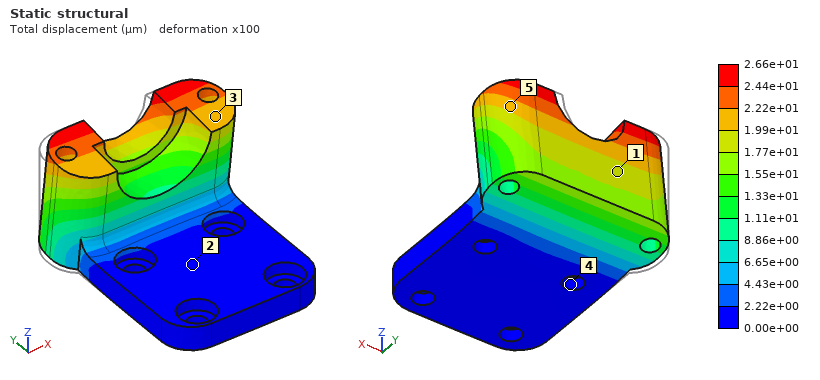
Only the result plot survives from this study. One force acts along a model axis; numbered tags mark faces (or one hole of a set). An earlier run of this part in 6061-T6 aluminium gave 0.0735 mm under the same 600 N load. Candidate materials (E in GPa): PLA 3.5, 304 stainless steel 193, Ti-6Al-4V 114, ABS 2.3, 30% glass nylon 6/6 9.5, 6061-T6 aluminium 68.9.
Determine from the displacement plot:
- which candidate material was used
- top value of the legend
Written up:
304 stainless steel
2.66e+01 µm
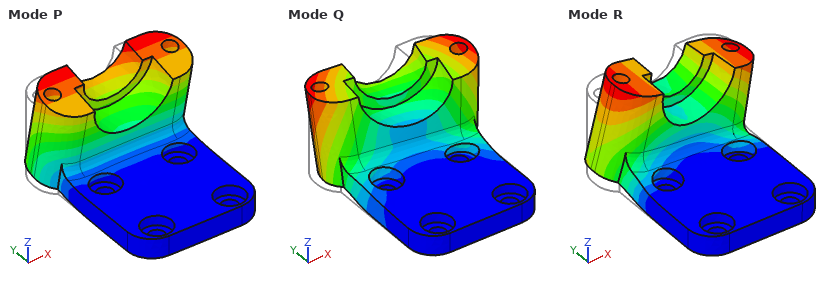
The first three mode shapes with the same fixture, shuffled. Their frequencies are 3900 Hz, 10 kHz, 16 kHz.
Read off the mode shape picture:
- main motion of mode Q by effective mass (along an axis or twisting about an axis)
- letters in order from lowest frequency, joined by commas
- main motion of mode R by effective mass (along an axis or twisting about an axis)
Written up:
along X
P, R, Q
along X
